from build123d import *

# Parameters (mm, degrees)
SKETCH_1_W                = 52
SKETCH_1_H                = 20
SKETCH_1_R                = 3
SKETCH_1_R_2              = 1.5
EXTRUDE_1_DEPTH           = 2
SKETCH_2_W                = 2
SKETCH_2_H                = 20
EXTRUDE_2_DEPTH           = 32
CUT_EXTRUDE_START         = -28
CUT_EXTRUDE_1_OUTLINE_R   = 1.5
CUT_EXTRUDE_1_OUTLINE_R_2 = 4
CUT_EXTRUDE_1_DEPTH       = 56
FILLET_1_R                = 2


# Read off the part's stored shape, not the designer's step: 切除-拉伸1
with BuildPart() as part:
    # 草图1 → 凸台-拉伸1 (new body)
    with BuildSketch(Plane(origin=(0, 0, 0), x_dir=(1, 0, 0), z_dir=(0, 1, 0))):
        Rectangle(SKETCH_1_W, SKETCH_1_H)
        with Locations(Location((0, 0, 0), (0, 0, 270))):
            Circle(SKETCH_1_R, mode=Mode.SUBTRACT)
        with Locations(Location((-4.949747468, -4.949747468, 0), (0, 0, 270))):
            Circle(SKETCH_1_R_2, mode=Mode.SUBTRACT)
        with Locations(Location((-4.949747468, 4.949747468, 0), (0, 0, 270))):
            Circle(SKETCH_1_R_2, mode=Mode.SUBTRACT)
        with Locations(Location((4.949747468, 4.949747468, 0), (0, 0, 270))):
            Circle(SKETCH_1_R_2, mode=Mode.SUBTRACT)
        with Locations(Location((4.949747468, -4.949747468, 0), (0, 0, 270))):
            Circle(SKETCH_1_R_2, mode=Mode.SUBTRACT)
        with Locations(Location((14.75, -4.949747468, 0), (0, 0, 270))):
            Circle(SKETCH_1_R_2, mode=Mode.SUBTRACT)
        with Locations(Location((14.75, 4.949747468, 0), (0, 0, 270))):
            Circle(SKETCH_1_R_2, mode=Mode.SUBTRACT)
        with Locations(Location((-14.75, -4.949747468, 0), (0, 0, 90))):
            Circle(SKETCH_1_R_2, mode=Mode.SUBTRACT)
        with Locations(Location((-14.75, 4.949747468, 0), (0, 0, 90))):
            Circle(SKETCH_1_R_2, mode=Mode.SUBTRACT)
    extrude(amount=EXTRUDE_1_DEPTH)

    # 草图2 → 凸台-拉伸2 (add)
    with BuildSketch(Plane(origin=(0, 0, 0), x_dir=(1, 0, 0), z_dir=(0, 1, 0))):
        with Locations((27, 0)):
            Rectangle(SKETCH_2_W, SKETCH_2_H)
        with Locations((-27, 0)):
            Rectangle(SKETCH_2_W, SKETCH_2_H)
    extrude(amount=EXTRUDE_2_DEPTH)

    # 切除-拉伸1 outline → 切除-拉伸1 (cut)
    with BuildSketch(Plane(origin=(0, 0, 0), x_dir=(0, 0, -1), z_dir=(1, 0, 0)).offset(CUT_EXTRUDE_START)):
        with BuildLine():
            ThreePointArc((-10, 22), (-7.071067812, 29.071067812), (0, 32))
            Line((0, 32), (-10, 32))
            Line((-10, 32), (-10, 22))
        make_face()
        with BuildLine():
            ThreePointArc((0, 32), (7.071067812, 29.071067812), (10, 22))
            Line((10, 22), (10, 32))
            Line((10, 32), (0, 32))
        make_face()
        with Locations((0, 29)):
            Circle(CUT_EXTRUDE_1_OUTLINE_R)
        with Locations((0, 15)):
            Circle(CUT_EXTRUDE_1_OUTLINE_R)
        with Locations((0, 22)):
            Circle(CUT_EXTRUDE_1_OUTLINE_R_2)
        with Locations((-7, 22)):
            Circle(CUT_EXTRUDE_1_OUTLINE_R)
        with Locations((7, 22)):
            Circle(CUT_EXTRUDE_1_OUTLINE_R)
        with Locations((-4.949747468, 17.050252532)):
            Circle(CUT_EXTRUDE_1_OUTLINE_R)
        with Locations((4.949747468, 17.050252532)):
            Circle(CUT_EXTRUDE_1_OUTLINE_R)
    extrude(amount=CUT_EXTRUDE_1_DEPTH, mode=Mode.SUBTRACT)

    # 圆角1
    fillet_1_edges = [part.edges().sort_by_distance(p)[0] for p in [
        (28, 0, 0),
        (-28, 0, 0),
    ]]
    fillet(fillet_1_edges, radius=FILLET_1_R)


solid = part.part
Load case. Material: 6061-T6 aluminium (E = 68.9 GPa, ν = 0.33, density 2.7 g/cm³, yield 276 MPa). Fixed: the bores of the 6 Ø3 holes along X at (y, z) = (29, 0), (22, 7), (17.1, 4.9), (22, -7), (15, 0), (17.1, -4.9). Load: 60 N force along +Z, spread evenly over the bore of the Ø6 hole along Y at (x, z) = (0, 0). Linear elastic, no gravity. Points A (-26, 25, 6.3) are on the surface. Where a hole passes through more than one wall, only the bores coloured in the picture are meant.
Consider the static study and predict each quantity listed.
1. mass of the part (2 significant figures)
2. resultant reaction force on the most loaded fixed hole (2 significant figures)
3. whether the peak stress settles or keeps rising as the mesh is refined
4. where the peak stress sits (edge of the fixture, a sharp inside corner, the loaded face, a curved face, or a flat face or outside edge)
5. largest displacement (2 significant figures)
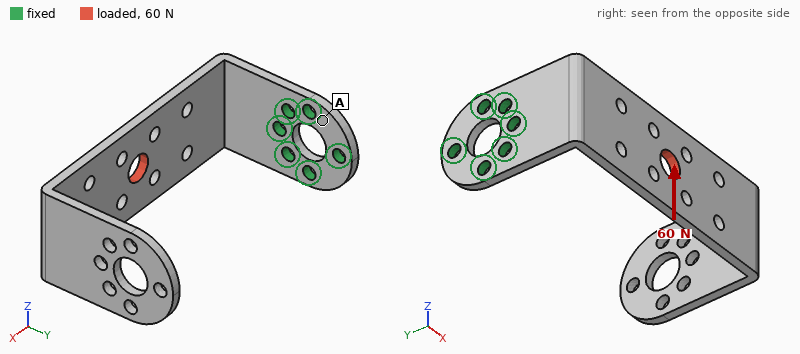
11 g
120 N
keeps rising
edge of the fixture
0.70 mm
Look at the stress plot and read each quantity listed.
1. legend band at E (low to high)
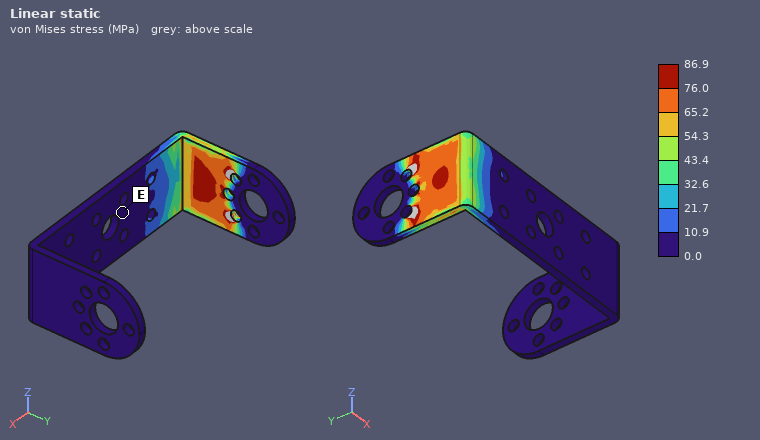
0.0 to 10.9 MPa
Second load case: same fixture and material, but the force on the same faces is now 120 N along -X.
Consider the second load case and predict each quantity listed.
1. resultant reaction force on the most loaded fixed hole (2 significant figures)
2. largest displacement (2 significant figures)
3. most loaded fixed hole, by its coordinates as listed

170 N
0.69 mm
(15, 0)
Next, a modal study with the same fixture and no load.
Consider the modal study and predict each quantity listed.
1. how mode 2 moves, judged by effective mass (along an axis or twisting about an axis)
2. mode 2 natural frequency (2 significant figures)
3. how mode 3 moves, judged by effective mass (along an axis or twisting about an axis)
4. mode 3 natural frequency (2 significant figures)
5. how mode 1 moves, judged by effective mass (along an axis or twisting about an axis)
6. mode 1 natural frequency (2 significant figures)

along Z
470 Hz
along X
990 Hz
along Y
240 Hz
